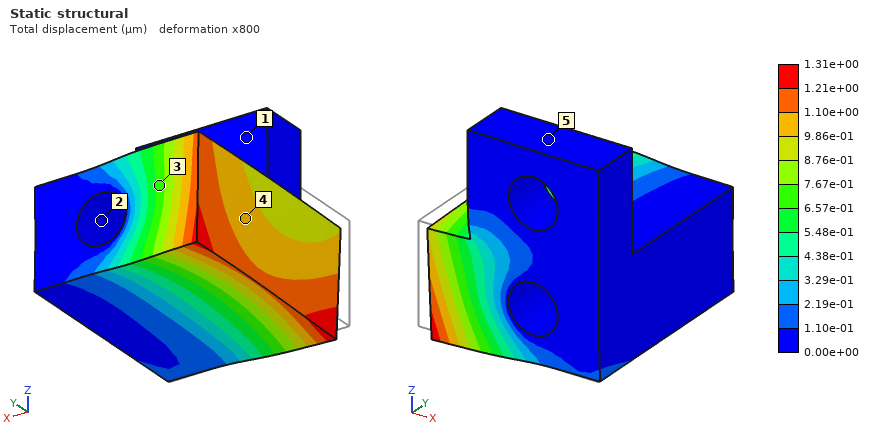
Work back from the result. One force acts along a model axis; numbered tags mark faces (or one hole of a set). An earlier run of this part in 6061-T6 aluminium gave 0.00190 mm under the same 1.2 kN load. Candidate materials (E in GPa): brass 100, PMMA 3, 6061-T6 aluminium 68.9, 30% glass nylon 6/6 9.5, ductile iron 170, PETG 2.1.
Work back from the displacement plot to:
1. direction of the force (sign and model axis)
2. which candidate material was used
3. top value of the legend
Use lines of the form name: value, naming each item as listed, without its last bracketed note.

direction of the force: +X
which candidate material was used: brass
top value of the legend: 1.31e+00 µm
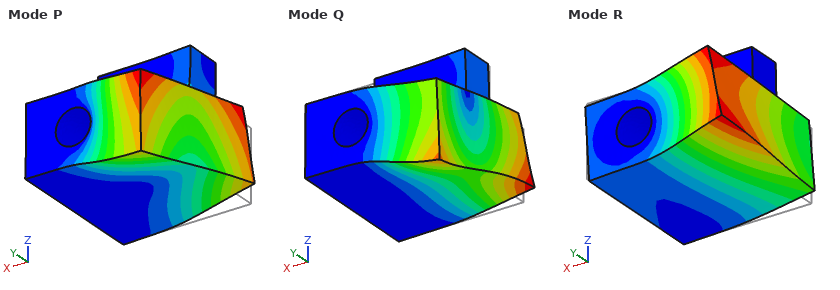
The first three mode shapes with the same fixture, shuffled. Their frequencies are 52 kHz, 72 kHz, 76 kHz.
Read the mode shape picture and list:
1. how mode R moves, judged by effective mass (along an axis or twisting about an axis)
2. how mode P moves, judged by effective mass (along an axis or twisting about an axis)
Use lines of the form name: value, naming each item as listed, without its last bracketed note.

how mode R moves, judged by effective mass: along Z
how mode P moves, judged by effective mass: along Y
